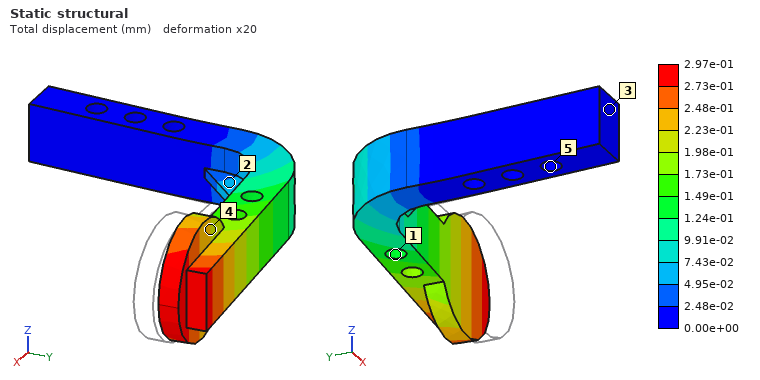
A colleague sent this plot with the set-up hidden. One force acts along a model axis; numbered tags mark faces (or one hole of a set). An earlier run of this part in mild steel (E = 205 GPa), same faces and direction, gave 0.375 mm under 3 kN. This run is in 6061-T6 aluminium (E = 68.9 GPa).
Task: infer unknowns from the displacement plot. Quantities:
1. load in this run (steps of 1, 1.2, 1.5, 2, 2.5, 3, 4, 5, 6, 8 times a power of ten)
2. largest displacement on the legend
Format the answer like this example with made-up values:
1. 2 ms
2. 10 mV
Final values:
1. 800 N
2. 2.97e-01 mm
